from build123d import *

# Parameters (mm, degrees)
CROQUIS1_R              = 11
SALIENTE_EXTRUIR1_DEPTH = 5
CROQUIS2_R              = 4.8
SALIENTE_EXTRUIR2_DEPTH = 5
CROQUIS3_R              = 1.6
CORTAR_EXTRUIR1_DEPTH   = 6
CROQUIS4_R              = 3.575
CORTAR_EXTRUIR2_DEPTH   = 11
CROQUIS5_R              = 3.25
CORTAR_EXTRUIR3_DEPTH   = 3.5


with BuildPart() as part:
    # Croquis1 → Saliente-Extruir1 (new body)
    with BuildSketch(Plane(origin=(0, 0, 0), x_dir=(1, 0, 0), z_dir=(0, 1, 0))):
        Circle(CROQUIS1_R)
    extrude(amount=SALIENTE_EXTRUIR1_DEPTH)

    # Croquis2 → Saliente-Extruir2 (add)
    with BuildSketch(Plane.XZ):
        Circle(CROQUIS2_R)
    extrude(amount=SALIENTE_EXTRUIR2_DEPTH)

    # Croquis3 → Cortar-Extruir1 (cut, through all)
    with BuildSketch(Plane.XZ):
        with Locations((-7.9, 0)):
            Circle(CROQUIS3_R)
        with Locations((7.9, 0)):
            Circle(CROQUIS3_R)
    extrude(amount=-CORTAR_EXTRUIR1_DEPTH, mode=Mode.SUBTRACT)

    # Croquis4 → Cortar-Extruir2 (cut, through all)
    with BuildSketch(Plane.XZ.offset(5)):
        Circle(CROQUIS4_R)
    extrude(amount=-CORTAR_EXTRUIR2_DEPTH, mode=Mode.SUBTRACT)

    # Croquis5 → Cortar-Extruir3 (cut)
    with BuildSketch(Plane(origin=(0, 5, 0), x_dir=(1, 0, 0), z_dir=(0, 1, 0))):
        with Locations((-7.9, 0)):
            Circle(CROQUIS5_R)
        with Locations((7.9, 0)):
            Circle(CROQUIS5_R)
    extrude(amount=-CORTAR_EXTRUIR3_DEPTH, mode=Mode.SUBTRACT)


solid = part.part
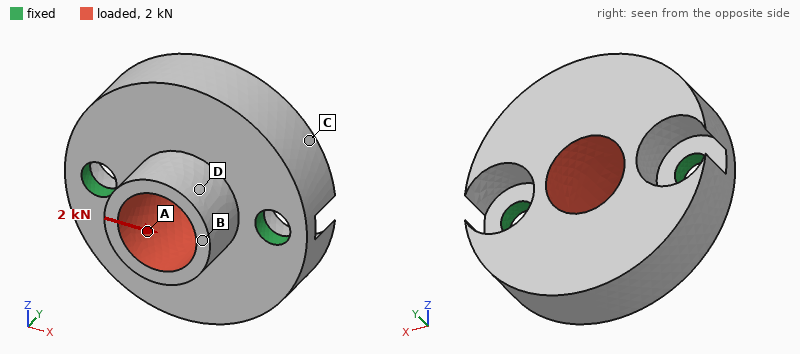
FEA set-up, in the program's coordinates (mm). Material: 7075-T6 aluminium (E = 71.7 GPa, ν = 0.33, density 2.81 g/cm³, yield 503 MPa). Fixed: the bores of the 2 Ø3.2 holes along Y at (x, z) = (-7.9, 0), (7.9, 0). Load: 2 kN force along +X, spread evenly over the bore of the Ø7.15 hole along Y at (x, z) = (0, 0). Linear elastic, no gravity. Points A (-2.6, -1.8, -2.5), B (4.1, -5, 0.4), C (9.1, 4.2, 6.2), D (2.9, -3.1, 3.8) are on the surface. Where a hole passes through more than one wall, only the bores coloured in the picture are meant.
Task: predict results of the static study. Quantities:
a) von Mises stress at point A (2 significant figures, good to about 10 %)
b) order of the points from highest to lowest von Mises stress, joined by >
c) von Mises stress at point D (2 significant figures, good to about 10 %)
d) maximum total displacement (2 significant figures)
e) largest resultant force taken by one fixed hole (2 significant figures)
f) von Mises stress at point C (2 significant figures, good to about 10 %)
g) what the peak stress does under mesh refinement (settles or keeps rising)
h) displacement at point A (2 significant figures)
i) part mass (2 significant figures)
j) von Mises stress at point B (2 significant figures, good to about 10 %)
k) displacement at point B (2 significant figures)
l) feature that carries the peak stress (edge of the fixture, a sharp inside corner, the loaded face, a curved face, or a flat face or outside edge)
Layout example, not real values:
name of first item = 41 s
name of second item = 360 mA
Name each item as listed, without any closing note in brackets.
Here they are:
von Mises stress at point A = 64 MPa
order of the points from highest to lowest von Mises stress, joined by > = A > B > D > C
von Mises stress at point D = 28 MPa
maximum total displacement = 16 µm
largest resultant force taken by one fixed hole = 1.0 kN
von Mises stress at point C = 13 MPa
what the peak stress does under mesh refinement = keeps rising
displacement at point A = 9.1 µm
part mass = 4.5 g
von Mises stress at point B = 45 MPa
displacement at point B = 16 µm
feature that carries the peak stress = edge of the fixture
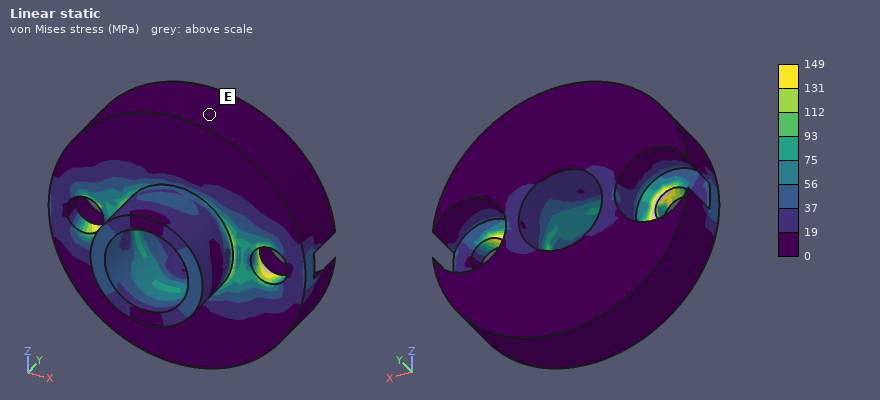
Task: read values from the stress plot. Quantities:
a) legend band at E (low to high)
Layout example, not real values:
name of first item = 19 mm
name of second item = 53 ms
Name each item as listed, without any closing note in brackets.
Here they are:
legend band at E = 0 to 19 MPa
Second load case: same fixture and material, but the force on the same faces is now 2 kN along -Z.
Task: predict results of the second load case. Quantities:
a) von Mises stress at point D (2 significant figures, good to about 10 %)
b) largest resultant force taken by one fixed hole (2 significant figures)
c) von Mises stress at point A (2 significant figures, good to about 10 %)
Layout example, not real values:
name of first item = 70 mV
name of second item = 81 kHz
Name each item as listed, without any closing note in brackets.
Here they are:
von Mises stress at point D = 27 MPa
largest resultant force taken by one fixed hole = 1.0 kN
von Mises stress at point A = 58 MPa
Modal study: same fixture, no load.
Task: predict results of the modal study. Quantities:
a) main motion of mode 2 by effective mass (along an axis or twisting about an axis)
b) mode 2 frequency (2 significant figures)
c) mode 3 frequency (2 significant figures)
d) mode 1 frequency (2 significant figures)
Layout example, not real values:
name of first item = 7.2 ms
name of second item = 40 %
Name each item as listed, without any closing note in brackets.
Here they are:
main motion of mode 2 by effective mass = along Y
mode 2 frequency = 23 kHz
mode 3 frequency = 41 kHz
mode 1 frequency = 10 kHz
